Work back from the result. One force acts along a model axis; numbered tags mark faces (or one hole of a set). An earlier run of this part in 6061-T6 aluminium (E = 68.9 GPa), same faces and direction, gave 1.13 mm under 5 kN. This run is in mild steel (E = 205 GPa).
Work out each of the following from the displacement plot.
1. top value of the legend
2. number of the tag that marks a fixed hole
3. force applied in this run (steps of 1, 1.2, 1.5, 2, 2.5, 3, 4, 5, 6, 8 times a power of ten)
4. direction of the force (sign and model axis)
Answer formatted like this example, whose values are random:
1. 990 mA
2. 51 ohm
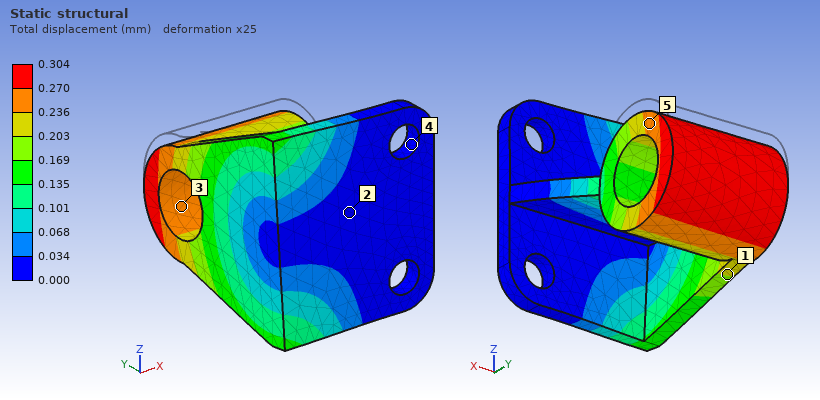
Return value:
1. 0.304 mm
2. 4
3. 4 kN
4. -Z
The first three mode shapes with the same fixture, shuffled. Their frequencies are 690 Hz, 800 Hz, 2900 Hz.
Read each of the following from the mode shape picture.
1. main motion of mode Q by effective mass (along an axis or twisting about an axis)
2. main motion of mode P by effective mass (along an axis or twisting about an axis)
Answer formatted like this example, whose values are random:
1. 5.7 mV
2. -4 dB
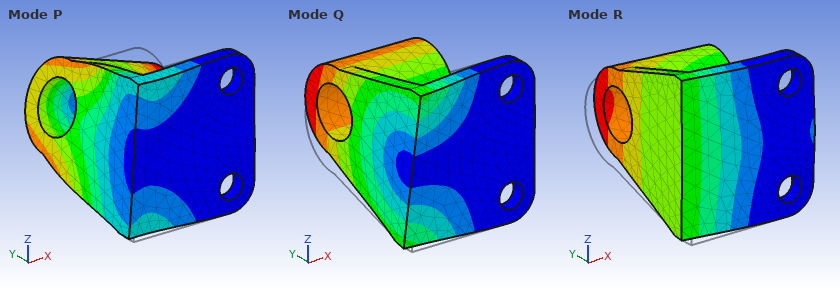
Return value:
1. along Z
2. twisting about Y
